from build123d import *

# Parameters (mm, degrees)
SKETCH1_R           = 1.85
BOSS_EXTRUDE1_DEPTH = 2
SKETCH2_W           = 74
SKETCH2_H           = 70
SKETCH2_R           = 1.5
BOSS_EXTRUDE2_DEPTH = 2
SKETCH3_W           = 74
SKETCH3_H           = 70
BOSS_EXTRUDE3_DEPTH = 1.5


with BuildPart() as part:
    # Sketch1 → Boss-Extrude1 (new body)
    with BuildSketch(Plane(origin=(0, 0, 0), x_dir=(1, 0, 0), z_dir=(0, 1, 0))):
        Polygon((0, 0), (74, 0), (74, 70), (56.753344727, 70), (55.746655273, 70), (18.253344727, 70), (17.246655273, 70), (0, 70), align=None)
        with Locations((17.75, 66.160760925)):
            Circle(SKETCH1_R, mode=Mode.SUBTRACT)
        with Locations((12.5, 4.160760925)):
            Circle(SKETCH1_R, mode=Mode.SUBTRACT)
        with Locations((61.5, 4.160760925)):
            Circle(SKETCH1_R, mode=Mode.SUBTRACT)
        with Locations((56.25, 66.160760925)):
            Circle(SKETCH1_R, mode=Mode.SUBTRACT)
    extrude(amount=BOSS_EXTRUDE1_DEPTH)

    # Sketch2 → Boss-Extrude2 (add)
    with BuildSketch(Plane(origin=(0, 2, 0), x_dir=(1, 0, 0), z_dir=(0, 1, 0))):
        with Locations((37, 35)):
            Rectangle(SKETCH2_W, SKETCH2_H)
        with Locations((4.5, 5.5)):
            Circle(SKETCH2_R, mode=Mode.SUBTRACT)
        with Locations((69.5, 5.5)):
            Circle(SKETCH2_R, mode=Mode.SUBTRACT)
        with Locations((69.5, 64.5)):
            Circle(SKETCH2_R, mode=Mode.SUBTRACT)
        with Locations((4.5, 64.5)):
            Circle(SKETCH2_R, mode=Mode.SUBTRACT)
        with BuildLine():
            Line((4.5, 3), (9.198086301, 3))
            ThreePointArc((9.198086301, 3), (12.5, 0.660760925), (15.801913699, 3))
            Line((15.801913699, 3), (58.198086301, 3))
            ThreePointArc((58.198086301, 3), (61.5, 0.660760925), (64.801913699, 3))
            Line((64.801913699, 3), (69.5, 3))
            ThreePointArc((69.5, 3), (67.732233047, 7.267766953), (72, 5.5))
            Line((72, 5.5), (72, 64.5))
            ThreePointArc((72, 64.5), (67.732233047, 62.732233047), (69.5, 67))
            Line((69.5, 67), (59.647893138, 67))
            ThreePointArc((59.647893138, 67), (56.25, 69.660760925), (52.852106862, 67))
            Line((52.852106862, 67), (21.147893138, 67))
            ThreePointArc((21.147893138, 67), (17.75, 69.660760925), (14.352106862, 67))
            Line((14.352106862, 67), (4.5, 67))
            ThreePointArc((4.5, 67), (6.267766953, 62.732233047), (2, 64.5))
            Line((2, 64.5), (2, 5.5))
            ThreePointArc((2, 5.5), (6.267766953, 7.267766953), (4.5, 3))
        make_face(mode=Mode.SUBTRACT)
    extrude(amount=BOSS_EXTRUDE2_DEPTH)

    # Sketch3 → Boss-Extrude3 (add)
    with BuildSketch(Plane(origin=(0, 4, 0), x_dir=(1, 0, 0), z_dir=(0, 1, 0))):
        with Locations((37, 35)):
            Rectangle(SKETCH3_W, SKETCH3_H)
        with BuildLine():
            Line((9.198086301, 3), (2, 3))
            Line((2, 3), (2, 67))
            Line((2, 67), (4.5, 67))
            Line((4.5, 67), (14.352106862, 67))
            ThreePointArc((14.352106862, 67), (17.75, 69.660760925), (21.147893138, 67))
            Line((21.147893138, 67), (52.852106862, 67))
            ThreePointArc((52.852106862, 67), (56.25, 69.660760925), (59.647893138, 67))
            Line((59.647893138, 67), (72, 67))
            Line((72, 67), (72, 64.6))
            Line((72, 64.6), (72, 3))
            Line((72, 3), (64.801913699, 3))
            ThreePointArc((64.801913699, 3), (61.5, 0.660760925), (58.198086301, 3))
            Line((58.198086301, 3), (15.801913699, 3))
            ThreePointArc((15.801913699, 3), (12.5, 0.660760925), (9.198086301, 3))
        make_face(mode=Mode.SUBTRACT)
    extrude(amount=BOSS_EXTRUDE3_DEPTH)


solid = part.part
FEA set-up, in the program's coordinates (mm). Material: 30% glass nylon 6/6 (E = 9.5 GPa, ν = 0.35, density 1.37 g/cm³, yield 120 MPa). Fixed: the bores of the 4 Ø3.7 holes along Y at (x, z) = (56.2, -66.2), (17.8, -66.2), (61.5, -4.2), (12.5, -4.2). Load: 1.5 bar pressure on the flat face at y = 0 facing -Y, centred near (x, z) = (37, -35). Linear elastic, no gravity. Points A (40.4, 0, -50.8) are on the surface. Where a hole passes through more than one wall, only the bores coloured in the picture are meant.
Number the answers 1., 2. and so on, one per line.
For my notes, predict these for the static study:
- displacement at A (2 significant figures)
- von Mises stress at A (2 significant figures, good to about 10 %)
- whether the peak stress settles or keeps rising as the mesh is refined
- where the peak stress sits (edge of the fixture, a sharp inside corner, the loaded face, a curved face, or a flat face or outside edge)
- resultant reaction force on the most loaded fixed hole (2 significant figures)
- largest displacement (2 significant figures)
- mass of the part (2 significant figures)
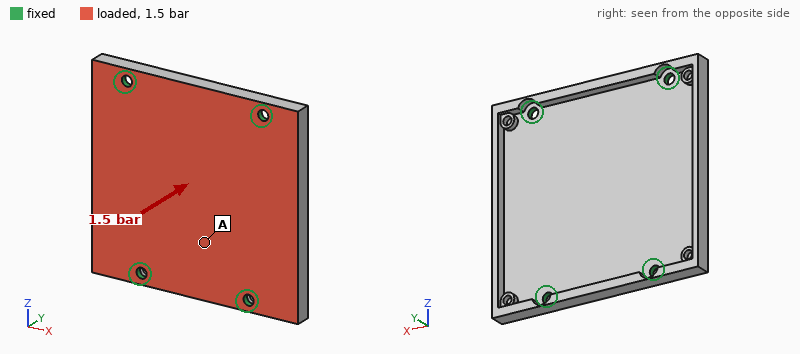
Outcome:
1. 0.63 mm
2. 16 MPa
3. keeps rising
4. edge of the fixture
5. 200 N
6. 1.0 mm
7. 17 g
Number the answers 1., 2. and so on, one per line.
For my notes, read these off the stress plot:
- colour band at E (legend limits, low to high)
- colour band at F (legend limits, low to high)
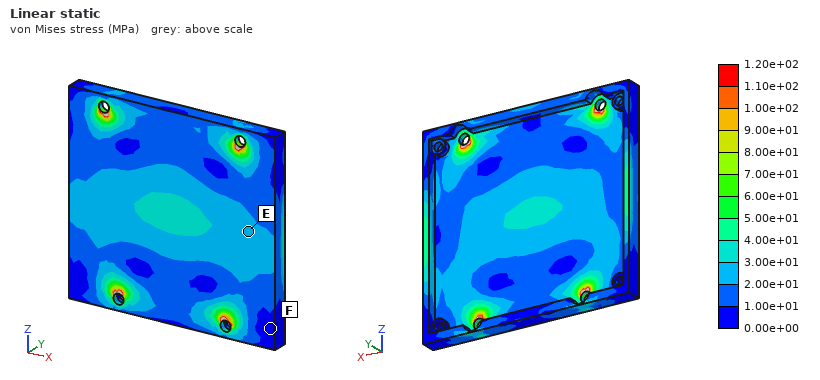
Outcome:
1. 2.00e+01 to 3.00e+01 MPa
2. 0.00e+00 to 1.00e+01 MPa
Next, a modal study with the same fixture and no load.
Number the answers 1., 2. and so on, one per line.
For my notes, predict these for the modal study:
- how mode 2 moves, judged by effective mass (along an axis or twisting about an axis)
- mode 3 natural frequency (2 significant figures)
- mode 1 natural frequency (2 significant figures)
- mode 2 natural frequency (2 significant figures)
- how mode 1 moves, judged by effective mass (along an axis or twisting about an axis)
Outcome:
1. twisting about Z
2. 2000 Hz
3. 1400 Hz
4. 1800 Hz
5. along Y
